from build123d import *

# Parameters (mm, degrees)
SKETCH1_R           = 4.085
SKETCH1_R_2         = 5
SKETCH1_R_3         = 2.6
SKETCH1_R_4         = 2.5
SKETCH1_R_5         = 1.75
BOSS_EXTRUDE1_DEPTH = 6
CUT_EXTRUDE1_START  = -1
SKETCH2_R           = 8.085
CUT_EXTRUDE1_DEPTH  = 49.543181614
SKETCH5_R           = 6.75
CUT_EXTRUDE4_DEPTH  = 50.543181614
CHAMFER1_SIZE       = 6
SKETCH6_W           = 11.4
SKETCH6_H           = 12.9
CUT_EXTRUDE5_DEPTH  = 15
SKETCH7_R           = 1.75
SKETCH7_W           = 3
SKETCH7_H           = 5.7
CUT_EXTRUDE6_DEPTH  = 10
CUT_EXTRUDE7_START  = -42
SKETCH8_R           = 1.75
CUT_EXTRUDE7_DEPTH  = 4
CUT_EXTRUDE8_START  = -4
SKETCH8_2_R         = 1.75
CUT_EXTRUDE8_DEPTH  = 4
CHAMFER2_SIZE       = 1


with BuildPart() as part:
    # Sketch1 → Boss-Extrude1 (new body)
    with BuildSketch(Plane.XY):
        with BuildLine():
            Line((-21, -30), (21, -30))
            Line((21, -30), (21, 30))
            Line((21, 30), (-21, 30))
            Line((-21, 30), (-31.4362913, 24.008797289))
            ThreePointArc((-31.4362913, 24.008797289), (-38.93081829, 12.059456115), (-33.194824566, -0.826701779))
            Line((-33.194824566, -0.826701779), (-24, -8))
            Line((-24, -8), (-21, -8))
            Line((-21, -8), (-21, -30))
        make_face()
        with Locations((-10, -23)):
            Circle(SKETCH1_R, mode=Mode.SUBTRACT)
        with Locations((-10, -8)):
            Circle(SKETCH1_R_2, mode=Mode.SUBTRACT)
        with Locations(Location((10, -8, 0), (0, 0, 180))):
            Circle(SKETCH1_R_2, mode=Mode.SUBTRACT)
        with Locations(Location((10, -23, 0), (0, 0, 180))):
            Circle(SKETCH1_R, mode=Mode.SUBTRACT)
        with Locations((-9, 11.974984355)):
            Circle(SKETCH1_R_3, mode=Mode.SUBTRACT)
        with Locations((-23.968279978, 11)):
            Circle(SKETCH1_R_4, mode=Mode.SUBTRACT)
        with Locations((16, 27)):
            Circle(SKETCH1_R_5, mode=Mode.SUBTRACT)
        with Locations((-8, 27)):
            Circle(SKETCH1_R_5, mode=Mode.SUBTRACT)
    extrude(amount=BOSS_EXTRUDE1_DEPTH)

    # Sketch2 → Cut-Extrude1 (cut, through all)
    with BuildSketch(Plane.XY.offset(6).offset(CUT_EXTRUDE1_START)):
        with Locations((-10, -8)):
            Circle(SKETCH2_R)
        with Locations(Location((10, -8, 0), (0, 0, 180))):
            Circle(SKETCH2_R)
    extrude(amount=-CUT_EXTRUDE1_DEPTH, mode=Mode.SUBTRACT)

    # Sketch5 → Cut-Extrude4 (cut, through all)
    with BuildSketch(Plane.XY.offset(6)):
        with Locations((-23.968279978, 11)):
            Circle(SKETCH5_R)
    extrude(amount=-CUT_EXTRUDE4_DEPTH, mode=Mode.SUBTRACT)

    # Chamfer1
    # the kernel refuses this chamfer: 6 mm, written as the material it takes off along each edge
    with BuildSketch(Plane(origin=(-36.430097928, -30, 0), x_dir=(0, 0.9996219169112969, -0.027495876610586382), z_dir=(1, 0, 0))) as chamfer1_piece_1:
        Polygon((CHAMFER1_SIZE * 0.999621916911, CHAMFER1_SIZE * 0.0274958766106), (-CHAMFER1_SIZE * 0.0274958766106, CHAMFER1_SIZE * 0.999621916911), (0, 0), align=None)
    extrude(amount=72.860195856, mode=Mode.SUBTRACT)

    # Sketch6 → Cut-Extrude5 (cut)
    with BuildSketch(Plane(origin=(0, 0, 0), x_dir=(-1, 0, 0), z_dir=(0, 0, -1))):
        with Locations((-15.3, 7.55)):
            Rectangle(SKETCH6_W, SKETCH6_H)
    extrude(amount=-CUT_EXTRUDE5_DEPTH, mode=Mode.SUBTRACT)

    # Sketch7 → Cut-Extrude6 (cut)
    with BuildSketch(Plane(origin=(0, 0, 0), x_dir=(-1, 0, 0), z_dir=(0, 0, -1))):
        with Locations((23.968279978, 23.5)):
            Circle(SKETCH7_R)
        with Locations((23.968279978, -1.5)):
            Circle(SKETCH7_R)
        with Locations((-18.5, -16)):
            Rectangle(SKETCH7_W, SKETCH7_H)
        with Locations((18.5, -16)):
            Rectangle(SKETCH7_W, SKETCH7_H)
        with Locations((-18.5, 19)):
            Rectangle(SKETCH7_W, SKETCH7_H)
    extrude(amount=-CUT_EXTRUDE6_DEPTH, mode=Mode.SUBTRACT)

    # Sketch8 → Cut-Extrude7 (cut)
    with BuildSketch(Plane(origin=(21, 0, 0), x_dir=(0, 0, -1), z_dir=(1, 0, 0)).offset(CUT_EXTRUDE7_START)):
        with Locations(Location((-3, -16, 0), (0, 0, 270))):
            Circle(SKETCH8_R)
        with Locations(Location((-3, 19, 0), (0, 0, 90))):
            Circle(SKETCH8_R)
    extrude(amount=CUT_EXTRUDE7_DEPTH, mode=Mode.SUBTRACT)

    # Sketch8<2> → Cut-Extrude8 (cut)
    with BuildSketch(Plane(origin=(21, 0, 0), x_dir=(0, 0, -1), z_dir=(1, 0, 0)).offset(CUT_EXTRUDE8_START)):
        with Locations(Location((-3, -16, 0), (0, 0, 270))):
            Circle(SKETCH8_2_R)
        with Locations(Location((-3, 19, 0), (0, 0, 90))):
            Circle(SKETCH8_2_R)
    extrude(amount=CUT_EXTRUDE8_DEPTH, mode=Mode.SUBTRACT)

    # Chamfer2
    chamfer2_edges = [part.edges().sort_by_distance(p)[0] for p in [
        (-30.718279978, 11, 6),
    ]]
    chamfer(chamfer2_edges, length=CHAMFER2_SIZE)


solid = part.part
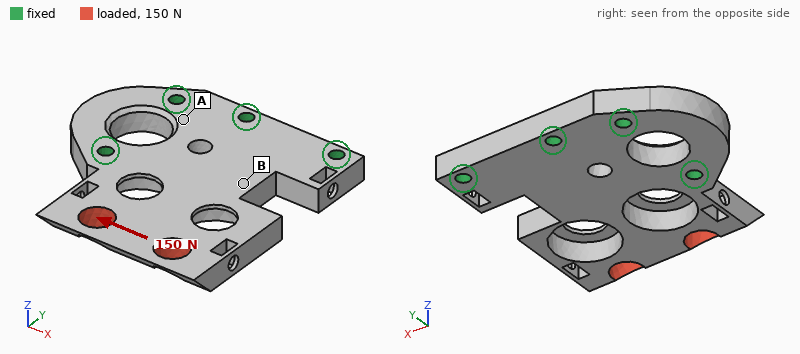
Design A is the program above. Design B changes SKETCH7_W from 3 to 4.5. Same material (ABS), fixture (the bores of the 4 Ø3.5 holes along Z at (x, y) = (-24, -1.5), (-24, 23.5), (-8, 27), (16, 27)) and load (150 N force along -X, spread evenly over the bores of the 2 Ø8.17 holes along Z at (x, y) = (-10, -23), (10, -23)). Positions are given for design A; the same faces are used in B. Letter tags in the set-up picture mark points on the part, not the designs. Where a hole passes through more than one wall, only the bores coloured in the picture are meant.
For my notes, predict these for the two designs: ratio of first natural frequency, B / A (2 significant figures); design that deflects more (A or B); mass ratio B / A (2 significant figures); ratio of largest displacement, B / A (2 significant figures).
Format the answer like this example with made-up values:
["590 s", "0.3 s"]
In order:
["0.99", "B", "0.99", "1.2"]
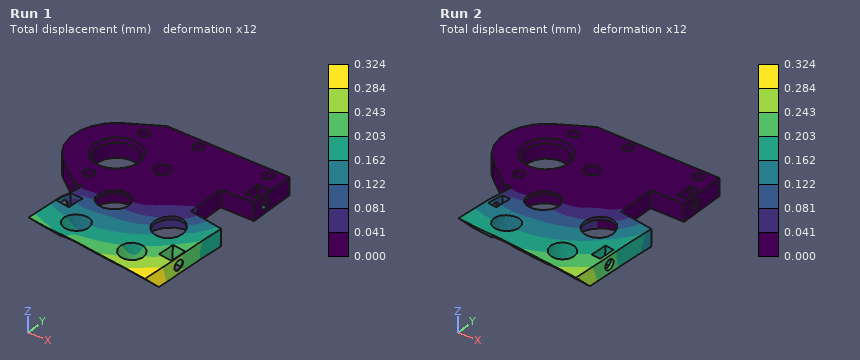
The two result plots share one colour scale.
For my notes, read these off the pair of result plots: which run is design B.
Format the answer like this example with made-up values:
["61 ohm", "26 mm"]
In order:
["Run 1"]
